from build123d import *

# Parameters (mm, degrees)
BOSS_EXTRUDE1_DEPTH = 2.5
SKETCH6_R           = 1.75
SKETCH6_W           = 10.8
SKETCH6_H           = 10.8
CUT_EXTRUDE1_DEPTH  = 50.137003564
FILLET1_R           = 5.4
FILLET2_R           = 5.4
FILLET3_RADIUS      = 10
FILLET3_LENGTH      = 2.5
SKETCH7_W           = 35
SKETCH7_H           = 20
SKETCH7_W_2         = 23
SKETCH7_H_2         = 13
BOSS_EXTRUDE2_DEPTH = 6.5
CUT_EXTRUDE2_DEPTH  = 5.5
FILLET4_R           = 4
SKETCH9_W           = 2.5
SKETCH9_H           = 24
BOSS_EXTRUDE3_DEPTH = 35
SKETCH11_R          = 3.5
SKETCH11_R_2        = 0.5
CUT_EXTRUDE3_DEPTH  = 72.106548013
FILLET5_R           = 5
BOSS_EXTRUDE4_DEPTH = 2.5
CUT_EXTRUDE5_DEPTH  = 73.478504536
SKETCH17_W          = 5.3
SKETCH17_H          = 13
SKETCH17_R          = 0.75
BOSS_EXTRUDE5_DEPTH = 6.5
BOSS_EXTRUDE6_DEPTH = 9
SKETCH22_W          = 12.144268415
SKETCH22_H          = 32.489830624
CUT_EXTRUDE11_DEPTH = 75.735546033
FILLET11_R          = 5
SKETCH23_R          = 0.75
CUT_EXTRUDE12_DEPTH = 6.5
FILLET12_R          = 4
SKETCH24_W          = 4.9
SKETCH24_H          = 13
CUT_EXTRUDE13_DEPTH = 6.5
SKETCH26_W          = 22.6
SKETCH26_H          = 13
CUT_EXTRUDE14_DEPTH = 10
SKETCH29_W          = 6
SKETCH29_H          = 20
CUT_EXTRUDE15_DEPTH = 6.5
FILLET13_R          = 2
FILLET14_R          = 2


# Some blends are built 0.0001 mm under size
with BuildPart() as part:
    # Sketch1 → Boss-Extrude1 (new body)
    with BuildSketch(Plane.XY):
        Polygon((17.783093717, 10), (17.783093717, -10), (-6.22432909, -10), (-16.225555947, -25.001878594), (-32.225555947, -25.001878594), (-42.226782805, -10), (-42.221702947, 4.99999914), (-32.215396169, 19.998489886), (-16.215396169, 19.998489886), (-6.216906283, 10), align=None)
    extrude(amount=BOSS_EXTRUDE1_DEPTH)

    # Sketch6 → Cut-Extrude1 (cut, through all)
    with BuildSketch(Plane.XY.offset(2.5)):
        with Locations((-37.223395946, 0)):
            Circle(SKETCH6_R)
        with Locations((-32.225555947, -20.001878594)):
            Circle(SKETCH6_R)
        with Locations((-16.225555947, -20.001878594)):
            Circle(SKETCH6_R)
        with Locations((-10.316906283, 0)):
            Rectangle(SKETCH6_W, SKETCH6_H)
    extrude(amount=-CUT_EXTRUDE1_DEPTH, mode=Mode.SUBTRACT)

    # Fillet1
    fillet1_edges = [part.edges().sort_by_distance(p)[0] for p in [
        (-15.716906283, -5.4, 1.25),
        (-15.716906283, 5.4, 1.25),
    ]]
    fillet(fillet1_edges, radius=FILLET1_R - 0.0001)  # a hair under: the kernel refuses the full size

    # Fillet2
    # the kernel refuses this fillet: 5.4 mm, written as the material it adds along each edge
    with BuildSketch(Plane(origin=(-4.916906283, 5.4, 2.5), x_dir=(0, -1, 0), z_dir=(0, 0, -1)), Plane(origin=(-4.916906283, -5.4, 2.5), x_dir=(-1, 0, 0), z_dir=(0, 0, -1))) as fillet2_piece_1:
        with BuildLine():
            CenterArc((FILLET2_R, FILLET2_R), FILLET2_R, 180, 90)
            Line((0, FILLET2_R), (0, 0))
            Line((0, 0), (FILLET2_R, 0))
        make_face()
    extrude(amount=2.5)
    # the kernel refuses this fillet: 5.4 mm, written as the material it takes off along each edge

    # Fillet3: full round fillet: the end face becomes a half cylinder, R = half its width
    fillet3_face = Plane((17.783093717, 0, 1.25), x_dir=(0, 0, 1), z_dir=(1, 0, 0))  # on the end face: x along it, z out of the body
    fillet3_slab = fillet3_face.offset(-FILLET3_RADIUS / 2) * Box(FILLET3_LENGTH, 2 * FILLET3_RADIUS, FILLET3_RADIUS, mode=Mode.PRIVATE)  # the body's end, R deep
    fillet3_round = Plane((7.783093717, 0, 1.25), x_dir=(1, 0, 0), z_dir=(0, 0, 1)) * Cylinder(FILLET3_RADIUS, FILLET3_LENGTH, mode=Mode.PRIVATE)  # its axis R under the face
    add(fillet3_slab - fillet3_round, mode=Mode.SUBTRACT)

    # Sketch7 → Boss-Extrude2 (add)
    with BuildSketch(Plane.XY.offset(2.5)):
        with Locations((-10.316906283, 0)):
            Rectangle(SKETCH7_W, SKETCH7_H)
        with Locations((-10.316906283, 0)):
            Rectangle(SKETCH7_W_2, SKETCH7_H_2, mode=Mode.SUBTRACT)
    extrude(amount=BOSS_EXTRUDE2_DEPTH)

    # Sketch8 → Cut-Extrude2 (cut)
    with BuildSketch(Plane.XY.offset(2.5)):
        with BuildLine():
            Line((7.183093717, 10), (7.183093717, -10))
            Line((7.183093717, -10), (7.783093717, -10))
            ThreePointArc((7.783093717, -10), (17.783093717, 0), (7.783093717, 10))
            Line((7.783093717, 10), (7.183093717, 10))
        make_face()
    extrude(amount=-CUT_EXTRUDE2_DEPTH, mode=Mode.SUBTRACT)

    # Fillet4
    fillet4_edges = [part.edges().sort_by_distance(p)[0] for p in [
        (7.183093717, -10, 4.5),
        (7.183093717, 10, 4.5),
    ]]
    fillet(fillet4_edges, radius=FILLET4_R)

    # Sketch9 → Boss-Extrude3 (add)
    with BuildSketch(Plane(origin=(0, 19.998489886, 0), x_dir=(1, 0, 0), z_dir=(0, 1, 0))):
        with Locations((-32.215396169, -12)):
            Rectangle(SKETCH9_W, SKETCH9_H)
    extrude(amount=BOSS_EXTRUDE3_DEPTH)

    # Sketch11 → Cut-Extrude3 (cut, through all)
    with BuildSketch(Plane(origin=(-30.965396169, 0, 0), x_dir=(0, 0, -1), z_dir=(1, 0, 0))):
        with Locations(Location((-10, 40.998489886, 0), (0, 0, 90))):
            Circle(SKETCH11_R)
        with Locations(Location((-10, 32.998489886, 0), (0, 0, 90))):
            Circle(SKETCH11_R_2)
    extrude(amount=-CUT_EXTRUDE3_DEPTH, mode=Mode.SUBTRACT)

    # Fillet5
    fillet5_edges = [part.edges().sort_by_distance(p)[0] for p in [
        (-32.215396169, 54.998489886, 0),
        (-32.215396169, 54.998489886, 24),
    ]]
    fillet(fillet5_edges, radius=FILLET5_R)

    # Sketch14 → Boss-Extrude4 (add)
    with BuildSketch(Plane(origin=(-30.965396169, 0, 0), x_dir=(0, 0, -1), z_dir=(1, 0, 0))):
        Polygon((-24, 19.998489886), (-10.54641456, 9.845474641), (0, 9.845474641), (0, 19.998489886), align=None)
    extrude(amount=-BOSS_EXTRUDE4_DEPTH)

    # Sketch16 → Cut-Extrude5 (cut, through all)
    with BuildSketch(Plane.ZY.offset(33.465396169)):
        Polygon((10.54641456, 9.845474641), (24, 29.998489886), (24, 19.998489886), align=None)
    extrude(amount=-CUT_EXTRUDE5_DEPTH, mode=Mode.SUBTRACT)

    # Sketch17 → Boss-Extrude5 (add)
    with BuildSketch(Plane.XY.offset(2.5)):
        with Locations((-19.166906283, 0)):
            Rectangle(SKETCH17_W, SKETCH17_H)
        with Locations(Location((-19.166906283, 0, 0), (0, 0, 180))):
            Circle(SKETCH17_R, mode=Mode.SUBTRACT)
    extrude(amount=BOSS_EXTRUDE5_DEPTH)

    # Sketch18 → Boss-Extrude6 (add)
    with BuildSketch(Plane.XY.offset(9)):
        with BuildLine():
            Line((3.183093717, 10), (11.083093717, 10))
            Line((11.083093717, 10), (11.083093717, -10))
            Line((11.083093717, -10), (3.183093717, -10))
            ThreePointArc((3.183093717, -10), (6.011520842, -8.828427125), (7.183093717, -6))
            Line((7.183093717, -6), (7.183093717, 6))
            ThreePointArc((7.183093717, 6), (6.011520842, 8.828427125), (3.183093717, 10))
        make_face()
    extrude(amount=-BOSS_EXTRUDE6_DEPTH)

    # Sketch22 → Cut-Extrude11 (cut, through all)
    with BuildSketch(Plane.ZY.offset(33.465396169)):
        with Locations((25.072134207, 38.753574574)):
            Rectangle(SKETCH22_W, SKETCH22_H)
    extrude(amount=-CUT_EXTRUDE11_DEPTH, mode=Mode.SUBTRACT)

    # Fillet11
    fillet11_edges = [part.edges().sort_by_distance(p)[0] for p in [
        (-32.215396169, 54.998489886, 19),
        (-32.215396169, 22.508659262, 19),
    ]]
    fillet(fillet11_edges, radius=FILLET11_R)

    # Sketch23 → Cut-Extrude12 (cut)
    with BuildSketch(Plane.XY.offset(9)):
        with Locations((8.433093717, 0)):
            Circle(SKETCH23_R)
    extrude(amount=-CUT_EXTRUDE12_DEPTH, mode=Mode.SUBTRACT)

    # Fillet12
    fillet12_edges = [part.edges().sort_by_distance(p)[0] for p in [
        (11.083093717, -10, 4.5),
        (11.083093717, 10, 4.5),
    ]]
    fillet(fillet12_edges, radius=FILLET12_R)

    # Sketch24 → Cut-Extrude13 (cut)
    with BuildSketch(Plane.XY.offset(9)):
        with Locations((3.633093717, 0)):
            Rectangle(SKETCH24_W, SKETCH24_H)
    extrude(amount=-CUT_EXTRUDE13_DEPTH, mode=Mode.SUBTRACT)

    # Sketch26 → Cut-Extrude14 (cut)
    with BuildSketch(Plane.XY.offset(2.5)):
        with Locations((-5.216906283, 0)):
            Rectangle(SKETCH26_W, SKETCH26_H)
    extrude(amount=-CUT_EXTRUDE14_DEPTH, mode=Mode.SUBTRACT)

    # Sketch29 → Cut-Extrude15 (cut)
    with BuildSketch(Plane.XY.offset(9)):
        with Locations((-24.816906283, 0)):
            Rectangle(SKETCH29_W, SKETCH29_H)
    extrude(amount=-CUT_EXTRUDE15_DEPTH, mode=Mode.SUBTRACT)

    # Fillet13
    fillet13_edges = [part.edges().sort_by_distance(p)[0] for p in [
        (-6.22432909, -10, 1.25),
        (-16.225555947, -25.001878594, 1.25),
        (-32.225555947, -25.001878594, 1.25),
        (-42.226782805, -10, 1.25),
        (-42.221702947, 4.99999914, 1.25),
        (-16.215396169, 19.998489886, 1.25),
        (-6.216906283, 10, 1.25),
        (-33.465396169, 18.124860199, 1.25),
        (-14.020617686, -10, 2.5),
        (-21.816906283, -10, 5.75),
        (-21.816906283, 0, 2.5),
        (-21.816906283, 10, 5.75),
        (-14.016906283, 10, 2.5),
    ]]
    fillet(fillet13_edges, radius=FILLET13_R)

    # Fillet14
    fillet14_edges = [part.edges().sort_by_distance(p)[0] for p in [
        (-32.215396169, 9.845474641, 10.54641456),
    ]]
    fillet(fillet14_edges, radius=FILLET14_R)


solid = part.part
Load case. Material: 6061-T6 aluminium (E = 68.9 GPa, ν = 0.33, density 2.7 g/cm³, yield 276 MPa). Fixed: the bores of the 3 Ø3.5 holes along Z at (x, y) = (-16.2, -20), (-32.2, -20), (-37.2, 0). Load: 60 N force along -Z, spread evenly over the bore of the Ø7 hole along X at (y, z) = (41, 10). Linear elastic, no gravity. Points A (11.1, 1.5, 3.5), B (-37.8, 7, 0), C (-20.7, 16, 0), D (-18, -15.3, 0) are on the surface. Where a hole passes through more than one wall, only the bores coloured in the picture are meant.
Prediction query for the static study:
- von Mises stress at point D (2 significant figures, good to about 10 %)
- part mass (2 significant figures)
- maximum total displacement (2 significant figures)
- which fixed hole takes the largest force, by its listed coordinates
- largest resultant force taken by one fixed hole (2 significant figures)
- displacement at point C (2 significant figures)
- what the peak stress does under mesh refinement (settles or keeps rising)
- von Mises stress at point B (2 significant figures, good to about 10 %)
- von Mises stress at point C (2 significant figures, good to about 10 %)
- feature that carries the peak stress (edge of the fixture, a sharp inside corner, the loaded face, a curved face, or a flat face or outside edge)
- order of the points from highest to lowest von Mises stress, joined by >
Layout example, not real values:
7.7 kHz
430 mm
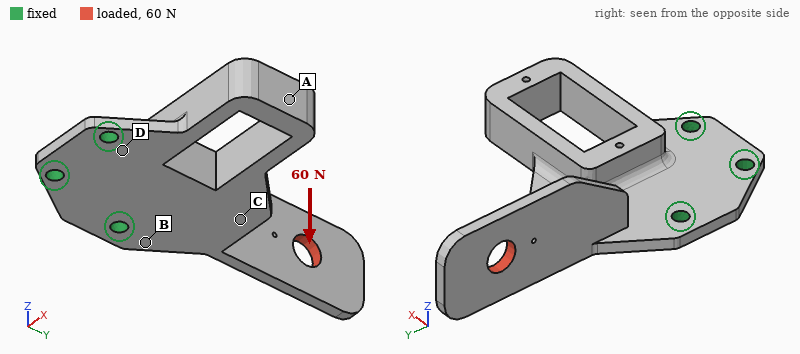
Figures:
20 MPa
20 g
0.55 mm
(-37.2, 0)
120 N
0.094 mm
keeps rising
72 MPa
38 MPa
edge of the fixture
B > C > D > A
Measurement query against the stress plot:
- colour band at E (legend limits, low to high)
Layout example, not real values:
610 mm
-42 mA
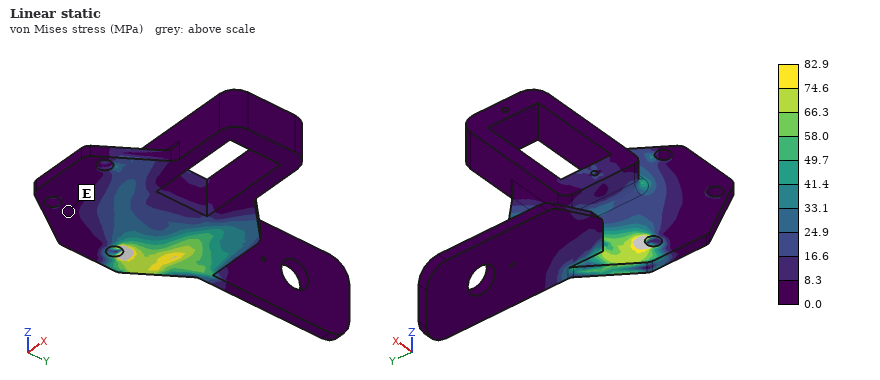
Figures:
0.0 to 8.3 MPa
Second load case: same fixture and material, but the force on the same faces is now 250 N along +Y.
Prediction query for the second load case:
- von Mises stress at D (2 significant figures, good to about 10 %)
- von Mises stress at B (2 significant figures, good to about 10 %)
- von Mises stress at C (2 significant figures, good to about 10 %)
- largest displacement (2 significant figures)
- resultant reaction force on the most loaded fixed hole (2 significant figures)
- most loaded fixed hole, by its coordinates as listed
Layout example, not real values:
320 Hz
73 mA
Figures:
17 MPa
67 MPa
43 MPa
0.57 mm
180 N
(-37.2, 0)
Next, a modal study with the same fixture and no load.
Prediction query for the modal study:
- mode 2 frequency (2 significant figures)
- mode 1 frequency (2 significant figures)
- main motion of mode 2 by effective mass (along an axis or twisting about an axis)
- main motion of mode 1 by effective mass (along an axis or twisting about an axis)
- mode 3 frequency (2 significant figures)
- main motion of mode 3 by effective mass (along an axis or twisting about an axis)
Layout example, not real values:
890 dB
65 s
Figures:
1100 Hz
950 Hz
along X
along Z
1700 Hz
along Z
